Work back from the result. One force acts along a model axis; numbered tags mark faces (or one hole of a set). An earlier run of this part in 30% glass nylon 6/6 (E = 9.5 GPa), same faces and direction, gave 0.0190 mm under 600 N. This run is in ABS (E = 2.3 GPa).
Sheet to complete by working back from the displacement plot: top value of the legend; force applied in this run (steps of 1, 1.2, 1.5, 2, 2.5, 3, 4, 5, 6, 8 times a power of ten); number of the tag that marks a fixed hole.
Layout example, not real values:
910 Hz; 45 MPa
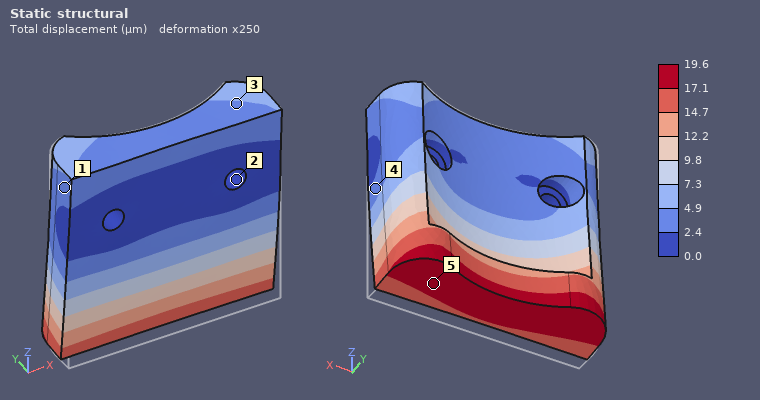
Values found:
19.6 µm; 150 N; 2
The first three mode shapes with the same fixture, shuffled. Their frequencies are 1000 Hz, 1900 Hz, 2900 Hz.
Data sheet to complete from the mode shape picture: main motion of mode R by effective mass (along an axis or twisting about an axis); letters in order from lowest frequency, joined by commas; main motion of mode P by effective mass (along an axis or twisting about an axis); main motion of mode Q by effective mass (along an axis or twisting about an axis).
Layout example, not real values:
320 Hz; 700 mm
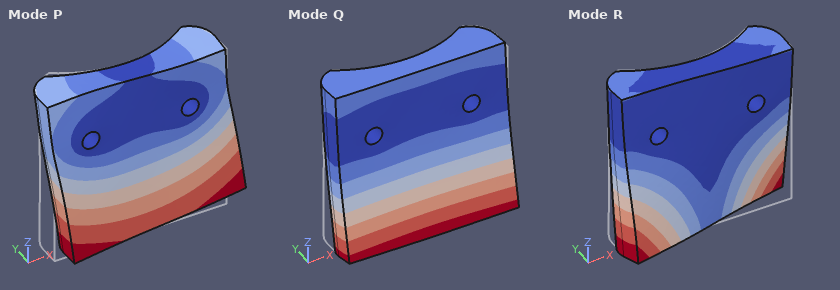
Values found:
twisting about Z; Q, R, P; along X; along Y
